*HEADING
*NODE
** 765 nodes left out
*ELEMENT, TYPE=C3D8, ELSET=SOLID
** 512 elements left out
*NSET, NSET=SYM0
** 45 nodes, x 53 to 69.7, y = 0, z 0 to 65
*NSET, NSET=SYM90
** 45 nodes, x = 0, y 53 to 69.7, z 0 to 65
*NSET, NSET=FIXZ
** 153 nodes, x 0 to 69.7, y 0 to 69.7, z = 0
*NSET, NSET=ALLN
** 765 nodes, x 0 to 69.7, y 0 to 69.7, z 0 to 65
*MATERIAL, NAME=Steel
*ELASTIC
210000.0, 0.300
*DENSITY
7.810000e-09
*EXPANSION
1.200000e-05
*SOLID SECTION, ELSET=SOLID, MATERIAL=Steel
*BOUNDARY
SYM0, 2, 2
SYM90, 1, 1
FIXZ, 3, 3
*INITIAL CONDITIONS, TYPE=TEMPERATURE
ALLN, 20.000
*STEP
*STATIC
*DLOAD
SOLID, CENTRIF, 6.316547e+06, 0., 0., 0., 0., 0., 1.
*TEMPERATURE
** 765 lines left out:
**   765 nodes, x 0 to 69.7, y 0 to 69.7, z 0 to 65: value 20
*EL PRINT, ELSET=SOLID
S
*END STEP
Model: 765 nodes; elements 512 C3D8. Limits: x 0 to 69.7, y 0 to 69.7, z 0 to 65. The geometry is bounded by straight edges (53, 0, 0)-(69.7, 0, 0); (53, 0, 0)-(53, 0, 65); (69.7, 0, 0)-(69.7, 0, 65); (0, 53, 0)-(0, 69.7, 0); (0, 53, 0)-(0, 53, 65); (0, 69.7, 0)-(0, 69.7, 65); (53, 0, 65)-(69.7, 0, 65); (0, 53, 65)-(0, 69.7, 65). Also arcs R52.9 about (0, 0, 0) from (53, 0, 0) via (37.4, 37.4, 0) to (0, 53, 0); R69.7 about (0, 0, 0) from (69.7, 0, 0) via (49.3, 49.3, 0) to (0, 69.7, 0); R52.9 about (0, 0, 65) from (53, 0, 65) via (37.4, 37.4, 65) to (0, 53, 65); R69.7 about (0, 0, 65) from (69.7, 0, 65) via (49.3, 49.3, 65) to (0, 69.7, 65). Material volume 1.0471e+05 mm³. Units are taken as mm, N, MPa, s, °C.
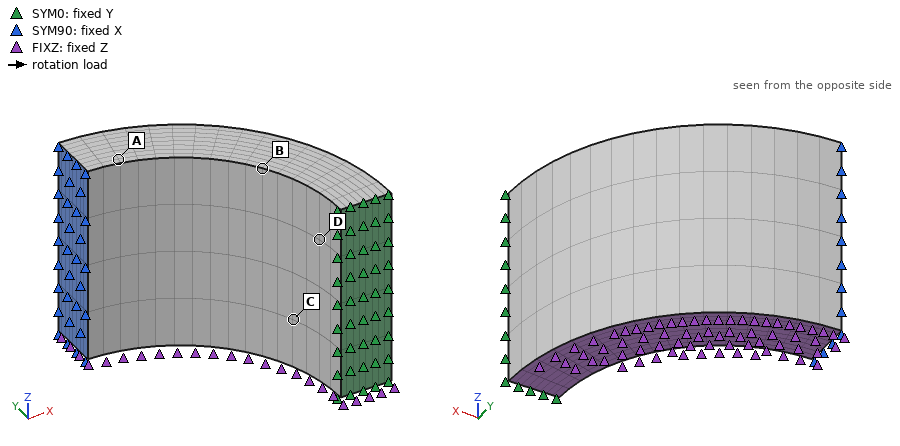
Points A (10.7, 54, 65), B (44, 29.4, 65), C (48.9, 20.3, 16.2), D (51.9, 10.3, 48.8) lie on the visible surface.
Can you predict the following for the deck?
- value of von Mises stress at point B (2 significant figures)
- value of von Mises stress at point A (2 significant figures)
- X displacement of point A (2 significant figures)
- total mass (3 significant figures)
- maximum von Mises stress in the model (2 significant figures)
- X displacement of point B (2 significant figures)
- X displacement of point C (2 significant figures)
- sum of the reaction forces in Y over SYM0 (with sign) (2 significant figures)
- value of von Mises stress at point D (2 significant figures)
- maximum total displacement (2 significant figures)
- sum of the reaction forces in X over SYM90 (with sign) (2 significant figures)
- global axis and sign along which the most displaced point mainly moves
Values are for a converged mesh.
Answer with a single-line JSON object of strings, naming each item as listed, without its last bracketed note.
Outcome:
{"value of von Mises stress at point B": "210 MPa", "value of von Mises stress at point A": "200 MPa", "X displacement of point A": "0.010 mm", "total mass": "0.818 kg", "maximum von Mises stress in the model": "220 MPa", "X displacement of point B": "0.045 mm", "X displacement of point C": "0.052 mm", "sum of the reaction forces in Y over SYM0 (with sign)": "-2.0e+05 N", "value of von Mises stress at point D": "220 MPa", "maximum total displacement": "0.057 mm", "sum of the reaction forces in X over SYM90 (with sign)": "-2.0e+05 N", "global axis and sign along which the most displaced point mainly moves": "+X"}
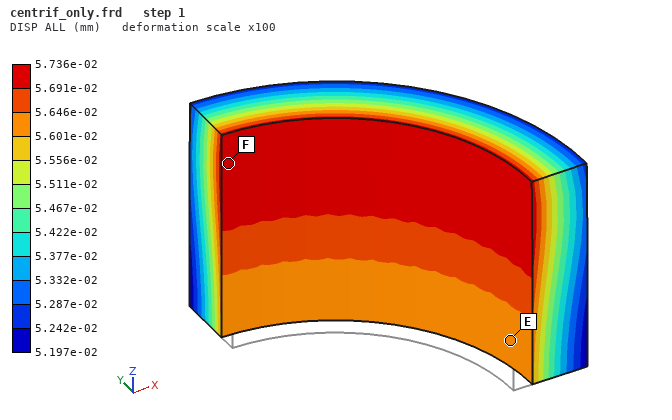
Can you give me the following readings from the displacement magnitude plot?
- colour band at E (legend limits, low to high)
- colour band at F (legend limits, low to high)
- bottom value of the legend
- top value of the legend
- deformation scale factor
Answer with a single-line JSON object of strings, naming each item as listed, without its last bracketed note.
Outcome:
{"colour band at E": "5.601e-02 to 5.646e-02 mm", "colour band at F": "5.691e-02 to 5.736e-02 mm", "bottom value of the legend": "5.197e-02 mm", "top value of the legend": "5.736e-02 mm", "deformation scale factor": "100"}
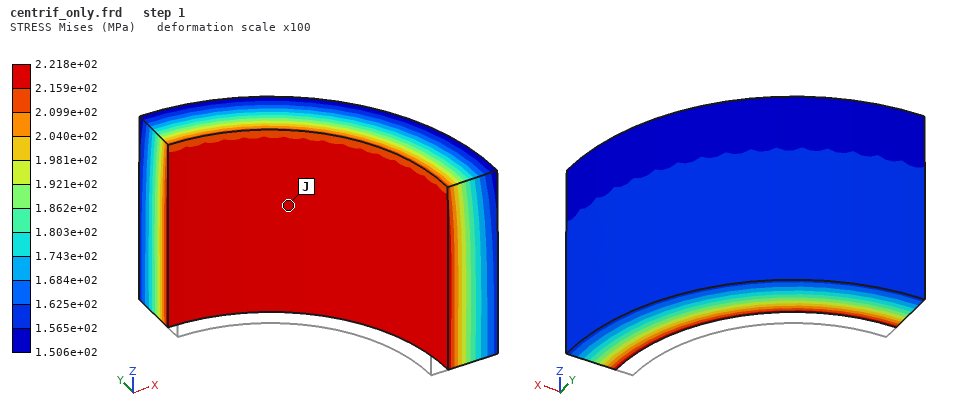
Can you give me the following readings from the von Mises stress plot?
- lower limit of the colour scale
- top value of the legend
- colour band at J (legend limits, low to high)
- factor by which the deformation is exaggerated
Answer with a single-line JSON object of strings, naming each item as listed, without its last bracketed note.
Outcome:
{"lower limit of the colour scale": "1.506e+02 MPa", "top value of the legend": "2.218e+02 MPa", "colour band at J": "2.159e+02 to 2.218e+02 MPa", "factor by which the deformation is exaggerated": "100"}
